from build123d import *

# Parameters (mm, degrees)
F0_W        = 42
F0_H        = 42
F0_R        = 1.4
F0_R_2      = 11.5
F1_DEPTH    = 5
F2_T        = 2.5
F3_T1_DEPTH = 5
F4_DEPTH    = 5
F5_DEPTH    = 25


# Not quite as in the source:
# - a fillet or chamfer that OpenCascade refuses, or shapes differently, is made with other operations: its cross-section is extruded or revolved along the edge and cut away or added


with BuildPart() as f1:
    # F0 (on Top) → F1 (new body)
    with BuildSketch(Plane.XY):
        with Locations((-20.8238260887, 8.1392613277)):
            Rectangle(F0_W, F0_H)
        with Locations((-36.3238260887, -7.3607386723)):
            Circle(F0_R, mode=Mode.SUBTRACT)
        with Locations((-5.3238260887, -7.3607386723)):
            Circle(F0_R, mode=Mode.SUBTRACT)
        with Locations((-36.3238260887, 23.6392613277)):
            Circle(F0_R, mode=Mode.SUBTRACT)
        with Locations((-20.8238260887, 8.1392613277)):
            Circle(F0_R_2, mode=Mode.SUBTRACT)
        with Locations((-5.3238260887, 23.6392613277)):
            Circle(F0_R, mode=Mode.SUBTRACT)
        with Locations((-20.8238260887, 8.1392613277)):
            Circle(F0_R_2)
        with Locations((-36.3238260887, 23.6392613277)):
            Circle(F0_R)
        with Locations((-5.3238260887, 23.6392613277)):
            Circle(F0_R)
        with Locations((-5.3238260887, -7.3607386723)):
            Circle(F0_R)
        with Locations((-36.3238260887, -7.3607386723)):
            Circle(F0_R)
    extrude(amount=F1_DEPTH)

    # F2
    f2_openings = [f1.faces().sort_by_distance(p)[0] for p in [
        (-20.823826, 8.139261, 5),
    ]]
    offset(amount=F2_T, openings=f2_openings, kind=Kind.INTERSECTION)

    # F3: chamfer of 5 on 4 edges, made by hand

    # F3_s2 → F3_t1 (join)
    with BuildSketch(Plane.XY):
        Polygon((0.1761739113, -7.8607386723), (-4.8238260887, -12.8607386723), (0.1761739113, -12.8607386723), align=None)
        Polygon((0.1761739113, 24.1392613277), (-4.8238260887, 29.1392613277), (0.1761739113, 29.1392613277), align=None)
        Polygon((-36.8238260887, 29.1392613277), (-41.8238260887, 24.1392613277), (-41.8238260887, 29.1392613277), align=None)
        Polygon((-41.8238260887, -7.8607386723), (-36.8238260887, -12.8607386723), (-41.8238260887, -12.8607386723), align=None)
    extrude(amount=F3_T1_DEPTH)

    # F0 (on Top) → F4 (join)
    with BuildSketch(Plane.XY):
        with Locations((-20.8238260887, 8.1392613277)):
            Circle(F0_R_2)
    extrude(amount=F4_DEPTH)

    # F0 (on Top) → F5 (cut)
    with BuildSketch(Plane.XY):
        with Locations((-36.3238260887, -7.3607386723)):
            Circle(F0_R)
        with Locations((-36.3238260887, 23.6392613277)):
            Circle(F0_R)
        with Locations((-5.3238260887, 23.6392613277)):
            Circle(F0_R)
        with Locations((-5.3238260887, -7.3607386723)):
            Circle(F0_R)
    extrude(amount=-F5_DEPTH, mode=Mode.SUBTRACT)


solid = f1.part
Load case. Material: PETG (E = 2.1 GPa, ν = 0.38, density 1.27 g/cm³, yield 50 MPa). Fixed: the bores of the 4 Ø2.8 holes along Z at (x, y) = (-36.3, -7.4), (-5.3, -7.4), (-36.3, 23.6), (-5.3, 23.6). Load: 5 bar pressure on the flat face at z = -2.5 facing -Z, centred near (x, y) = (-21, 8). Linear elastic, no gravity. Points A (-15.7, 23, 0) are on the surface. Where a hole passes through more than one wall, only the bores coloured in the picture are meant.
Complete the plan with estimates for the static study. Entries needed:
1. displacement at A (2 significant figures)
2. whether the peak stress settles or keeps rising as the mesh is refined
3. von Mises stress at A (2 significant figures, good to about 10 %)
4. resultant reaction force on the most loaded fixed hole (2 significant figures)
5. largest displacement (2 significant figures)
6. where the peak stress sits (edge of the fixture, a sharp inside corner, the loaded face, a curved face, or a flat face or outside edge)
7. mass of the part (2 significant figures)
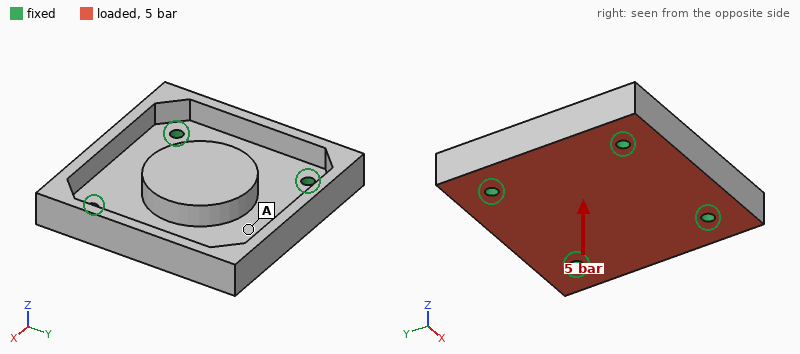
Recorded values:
0.26 mm
keeps rising
8.7 MPa
270 N
0.36 mm
edge of the fixture
13 g
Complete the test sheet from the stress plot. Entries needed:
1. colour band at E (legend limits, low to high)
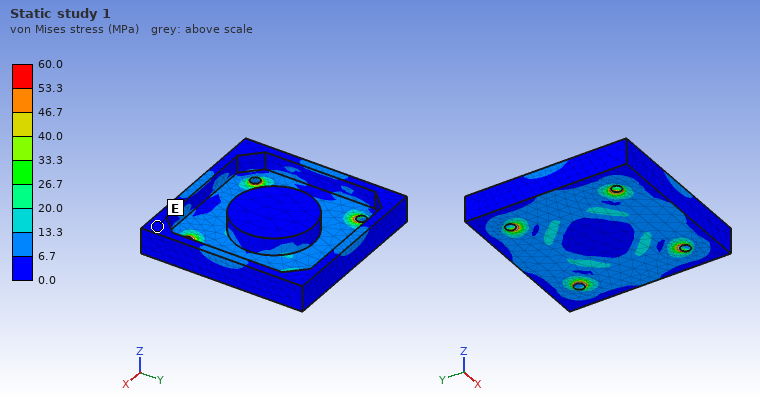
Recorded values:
0.0 to 6.7 MPa
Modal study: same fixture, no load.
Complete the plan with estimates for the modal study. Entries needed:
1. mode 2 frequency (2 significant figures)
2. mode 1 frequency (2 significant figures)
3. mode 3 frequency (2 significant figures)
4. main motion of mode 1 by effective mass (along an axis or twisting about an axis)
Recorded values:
3500 Hz
2600 Hz
3800 Hz
along Z
